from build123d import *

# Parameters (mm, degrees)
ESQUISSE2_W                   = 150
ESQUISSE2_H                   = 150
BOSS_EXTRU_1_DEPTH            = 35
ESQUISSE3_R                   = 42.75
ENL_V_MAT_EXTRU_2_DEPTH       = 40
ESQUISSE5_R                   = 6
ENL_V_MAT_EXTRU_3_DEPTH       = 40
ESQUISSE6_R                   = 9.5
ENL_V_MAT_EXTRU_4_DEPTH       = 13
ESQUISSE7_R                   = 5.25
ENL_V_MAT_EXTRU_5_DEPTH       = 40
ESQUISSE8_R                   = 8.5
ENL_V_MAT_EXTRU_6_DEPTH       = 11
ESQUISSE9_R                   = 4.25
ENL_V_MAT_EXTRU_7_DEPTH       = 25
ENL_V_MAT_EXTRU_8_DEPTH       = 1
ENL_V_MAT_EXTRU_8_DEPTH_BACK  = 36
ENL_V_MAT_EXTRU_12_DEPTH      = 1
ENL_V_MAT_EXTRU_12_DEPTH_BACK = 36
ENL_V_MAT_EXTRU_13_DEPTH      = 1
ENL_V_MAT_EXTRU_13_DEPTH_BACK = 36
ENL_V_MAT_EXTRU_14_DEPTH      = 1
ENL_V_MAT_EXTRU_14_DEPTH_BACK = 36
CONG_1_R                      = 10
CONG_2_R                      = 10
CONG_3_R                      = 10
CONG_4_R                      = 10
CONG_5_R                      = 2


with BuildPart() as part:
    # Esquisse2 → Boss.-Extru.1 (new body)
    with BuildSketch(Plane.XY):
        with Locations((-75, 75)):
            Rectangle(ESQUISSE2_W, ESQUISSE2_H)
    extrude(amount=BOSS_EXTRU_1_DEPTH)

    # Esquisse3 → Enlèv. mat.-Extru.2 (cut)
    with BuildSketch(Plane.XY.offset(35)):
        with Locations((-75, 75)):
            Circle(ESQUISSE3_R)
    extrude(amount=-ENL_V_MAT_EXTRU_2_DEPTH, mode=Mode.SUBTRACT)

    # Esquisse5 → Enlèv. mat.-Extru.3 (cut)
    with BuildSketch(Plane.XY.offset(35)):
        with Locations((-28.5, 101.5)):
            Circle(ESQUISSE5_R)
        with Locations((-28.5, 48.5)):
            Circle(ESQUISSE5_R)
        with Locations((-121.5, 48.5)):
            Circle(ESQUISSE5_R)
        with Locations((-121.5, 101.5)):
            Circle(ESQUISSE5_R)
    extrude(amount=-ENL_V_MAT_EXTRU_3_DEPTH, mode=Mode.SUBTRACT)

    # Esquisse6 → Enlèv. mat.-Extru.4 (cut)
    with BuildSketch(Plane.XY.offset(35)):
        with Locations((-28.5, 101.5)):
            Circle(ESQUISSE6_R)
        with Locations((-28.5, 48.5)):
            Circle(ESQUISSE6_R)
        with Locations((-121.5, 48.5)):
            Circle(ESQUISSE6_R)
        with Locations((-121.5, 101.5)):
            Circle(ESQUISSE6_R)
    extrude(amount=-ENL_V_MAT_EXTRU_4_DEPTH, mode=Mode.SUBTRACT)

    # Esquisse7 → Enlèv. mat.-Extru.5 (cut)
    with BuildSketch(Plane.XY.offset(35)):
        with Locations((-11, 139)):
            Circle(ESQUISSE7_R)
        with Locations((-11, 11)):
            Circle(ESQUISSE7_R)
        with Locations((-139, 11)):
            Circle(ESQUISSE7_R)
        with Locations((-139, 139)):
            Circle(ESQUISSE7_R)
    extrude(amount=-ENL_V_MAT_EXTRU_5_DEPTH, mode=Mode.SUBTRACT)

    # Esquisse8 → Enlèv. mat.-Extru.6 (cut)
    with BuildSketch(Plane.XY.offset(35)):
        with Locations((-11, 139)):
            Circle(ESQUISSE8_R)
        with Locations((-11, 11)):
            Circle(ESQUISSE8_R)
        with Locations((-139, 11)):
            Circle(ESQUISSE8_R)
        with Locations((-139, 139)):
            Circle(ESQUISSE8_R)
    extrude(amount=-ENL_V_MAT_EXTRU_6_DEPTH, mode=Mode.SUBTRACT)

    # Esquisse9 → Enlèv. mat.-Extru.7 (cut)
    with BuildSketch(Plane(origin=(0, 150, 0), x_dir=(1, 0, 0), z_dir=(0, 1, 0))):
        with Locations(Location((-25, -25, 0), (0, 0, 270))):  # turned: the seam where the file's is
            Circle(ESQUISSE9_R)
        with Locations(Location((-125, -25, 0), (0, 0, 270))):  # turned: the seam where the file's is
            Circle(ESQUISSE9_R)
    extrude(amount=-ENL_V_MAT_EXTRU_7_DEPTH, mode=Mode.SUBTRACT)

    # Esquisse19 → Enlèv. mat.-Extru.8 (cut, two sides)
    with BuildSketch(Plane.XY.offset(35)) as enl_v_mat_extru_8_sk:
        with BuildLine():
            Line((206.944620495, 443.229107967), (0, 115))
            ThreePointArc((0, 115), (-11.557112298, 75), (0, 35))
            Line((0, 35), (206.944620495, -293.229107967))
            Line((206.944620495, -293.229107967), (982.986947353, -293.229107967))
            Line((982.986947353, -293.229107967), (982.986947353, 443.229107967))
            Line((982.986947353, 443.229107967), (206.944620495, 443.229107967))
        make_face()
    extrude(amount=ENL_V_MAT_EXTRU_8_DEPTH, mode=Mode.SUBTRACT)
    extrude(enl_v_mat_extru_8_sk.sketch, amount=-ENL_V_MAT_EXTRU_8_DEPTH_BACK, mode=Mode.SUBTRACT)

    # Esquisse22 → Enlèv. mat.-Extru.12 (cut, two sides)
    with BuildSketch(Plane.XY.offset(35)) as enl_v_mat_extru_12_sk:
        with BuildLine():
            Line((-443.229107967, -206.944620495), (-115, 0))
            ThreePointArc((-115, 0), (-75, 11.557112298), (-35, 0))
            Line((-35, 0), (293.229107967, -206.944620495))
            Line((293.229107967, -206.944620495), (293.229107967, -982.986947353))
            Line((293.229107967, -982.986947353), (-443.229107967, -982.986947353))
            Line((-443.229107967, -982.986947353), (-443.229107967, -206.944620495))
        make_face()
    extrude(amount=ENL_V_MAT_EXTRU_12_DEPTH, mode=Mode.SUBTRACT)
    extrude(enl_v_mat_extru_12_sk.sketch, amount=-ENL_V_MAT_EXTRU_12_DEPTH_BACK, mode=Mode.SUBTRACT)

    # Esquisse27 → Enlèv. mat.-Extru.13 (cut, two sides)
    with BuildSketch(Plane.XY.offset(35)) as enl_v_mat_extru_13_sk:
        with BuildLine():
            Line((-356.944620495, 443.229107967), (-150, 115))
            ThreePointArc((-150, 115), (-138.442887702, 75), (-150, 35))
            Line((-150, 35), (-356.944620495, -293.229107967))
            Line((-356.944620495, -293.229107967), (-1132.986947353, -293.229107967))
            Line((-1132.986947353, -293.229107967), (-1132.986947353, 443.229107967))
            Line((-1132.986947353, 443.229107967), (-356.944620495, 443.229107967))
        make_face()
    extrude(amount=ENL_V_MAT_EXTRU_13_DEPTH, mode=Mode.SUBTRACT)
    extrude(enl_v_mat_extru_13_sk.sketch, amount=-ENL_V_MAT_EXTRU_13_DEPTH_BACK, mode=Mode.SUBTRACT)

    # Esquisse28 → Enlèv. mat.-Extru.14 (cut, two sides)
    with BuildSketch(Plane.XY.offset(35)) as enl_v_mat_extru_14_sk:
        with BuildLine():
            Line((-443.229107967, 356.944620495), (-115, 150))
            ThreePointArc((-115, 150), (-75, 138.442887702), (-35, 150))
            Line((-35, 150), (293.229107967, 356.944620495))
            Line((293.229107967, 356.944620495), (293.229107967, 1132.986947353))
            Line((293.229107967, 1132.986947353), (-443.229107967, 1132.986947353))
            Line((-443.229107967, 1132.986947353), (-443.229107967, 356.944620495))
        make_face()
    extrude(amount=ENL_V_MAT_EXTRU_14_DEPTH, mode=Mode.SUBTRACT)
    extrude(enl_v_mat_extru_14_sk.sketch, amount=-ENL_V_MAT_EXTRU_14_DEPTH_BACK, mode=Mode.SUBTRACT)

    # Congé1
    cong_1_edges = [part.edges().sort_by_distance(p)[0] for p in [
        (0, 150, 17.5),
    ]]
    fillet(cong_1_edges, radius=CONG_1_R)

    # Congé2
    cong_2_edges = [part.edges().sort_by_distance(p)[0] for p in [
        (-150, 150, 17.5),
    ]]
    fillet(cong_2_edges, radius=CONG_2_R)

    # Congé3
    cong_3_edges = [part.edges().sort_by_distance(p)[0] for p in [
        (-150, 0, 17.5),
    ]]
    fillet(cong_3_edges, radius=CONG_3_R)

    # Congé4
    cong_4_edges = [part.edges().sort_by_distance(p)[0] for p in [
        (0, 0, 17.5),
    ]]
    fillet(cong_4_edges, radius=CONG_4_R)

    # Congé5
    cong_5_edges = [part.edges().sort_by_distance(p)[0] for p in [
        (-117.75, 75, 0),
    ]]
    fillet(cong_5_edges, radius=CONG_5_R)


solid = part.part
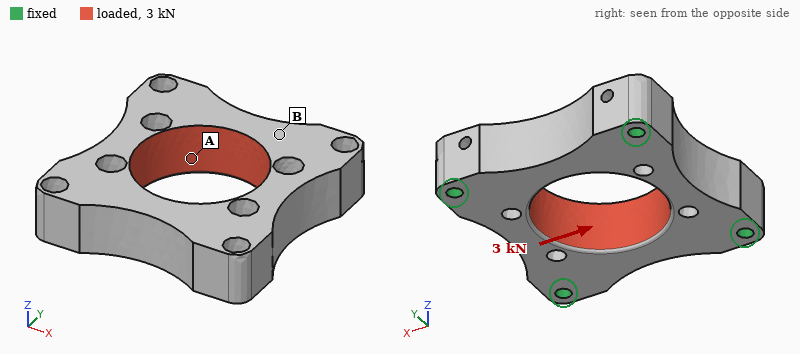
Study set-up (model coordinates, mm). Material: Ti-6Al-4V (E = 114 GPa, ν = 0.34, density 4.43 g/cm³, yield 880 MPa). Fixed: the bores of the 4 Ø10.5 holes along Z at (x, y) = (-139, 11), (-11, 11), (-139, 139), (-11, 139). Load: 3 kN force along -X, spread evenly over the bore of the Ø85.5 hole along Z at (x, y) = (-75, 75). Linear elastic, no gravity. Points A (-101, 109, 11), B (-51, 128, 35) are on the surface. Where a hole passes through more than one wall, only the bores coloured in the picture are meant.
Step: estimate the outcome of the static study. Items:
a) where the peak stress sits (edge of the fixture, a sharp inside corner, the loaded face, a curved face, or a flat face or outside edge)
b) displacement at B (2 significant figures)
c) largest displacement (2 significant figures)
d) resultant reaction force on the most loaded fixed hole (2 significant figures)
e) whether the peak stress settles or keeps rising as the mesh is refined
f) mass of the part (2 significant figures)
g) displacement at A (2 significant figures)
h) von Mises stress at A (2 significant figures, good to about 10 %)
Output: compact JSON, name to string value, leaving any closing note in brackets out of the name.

{"where the peak stress sits": "edge of the fixture", "displacement at B": "0.43 µm", "largest displacement": "1.4 µm", "resultant reaction force on the most loaded fixed hole": "860 N", "whether the peak stress settles or keeps rising as the mesh is refined": "keeps rising", "mass of the part": "2.0 kg", "displacement at A": "0.63 µm", "von Mises stress at A": "1.4 MPa"}
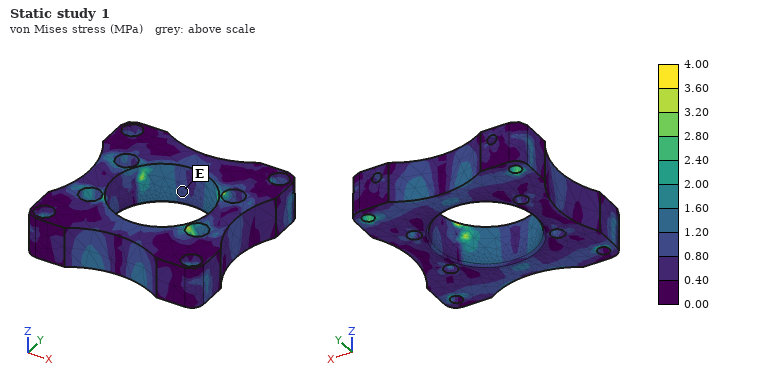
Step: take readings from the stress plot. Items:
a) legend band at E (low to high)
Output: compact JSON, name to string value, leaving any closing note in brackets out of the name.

{"legend band at E": "0.80 to 1.20 MPa"}
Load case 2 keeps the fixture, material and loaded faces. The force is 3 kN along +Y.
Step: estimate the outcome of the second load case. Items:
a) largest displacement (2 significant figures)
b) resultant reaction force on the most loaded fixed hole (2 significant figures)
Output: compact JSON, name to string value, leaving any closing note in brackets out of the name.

{"largest displacement": "1.3 µm", "resultant reaction force on the most loaded fixed hole": "870 N"}
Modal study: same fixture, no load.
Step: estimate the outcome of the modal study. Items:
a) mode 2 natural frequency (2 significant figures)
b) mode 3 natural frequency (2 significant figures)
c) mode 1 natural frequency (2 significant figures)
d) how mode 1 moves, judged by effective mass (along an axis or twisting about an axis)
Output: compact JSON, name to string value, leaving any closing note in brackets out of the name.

{"mode 2 natural frequency": "5900 Hz", "mode 3 natural frequency": "7100 Hz", "mode 1 natural frequency": "5500 Hz", "how mode 1 moves, judged by effective mass": "along Z"}
